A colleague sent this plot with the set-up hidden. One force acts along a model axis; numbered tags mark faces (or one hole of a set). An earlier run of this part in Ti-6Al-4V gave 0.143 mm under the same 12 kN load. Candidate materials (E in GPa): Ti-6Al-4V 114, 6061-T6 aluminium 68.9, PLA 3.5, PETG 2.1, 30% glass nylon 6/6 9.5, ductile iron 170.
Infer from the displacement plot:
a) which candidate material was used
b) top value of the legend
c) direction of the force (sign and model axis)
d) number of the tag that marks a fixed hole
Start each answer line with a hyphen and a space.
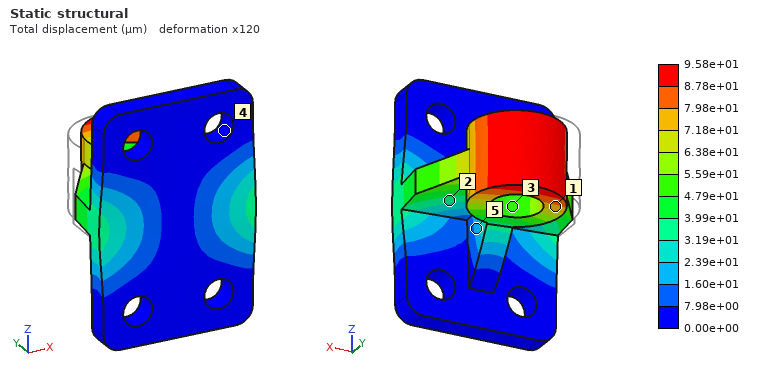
- ductile iron
- 9.58e+01 µm
- +X
- 4
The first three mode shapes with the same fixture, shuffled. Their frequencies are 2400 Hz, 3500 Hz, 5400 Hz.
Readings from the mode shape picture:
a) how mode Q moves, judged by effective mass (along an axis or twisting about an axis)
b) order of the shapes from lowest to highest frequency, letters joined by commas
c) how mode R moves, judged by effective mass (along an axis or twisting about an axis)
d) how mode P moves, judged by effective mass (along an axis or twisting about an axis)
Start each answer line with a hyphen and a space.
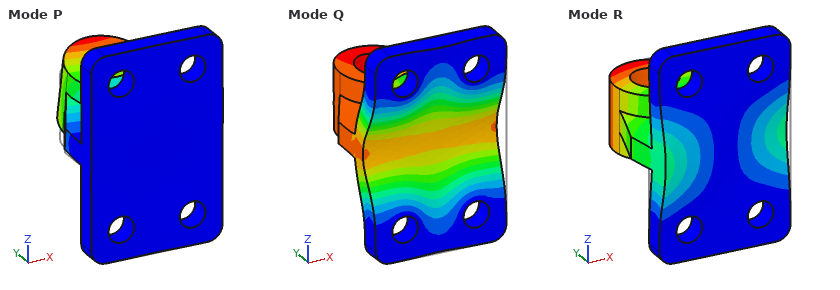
- along Y
- R, P, Q
- along X
- along Z
